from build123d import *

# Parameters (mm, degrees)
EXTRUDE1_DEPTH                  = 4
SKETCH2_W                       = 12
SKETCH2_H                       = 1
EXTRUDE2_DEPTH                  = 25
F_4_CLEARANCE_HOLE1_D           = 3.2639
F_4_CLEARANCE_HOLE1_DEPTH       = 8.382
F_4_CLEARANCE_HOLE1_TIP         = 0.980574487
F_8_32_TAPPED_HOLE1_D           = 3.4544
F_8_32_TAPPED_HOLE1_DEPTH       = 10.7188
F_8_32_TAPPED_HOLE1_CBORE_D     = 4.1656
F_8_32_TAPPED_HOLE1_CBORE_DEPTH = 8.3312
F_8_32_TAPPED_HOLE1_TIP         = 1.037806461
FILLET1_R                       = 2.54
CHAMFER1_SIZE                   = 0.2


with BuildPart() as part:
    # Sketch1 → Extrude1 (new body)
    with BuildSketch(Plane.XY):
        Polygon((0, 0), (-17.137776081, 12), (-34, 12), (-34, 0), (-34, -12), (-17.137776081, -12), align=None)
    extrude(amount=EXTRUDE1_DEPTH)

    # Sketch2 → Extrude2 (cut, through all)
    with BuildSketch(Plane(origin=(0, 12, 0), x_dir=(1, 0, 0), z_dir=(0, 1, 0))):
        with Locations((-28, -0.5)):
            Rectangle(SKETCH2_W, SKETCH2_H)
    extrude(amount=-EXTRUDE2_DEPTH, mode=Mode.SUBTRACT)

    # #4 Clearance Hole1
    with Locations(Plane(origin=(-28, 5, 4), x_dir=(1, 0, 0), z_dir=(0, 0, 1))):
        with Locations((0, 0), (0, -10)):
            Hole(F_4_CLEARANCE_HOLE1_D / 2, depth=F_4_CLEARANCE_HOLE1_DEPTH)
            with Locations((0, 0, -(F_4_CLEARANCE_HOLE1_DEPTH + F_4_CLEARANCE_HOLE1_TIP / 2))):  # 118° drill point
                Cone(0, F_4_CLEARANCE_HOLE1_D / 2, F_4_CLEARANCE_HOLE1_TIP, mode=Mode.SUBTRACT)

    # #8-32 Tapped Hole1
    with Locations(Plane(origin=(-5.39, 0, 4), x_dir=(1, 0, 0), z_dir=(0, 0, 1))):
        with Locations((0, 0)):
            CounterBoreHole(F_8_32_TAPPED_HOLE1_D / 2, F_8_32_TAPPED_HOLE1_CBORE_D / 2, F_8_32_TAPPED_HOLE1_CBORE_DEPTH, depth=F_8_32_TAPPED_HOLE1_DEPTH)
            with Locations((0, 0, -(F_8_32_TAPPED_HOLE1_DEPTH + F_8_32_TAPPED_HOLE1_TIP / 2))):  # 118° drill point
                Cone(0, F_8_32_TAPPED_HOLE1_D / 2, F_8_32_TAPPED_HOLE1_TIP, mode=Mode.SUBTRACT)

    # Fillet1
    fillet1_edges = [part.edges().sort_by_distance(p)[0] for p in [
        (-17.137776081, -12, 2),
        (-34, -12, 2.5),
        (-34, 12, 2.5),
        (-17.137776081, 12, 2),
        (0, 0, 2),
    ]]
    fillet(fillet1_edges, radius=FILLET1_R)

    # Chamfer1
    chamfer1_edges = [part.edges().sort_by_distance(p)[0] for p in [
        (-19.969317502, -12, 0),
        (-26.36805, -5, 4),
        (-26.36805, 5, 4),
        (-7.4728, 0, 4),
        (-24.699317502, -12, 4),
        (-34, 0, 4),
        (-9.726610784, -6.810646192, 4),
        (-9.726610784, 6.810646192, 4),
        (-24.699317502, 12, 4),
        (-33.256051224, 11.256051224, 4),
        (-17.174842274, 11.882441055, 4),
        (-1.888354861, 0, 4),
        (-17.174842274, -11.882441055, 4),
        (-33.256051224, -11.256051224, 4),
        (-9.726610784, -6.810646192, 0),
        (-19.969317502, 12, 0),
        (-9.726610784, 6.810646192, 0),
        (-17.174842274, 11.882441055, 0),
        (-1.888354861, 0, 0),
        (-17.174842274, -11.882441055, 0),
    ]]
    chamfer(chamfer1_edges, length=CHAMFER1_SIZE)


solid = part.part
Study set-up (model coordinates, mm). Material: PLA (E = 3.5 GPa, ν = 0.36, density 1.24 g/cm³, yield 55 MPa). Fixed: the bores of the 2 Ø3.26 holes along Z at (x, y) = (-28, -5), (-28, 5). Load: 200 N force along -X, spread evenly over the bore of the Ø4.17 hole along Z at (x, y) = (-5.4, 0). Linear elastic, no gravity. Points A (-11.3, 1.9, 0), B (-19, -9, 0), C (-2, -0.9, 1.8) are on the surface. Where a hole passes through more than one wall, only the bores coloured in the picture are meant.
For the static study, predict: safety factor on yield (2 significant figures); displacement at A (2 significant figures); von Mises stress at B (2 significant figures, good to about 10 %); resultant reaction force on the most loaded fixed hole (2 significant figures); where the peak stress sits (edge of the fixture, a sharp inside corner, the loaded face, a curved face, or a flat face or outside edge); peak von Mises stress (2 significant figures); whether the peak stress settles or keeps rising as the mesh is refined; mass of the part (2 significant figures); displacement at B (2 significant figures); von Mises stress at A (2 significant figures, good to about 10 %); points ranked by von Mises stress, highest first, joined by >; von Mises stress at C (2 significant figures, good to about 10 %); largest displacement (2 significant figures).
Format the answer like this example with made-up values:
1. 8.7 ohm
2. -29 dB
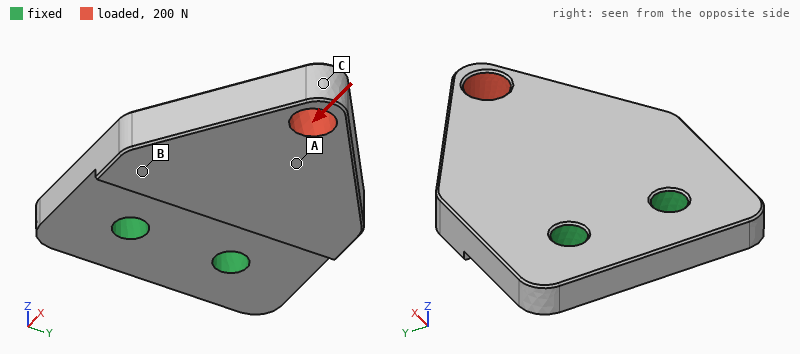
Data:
1. 3.0
2. 0.059 mm
3. 2.0 MPa
4. 100 N
5. the loaded face
6. 18 MPa
7. settles
8. 2.5 g
9. 0.027 mm
10. 4.6 MPa
11. C > A > B
12. 6.5 MPa
13. 0.11 mm
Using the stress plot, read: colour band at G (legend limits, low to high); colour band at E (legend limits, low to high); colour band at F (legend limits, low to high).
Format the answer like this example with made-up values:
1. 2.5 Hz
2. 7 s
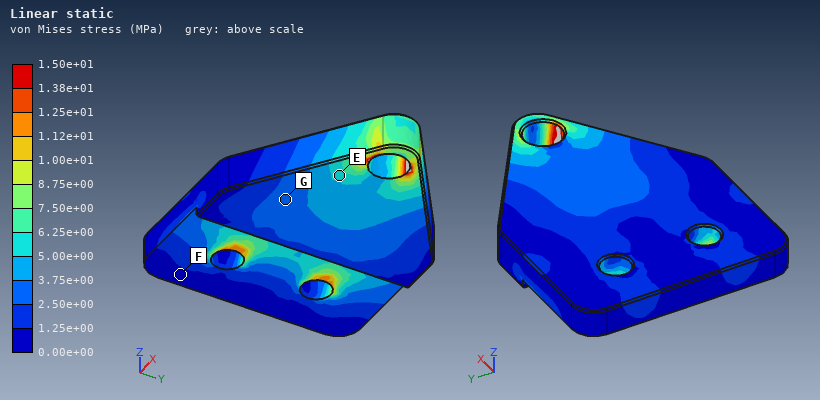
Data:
1. 2.50e+00 to 3.75e+00 MPa
2. 5.00e+00 to 6.25e+00 MPa
3. 0.00e+00 to 1.25e+00 MPa
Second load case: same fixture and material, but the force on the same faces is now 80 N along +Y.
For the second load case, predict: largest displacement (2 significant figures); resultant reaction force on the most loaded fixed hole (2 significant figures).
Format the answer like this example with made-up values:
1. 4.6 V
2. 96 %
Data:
1. 95 µm
2. 150 N
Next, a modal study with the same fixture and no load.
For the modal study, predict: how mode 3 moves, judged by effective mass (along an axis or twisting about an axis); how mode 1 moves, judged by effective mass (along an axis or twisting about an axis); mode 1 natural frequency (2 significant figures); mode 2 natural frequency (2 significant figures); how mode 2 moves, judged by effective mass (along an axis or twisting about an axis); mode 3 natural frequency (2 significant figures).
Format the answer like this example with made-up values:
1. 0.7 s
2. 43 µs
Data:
1. along Y
2. along Z
3. 1900 Hz
4. 5700 Hz
5. twisting about X
6. 7100 Hz
